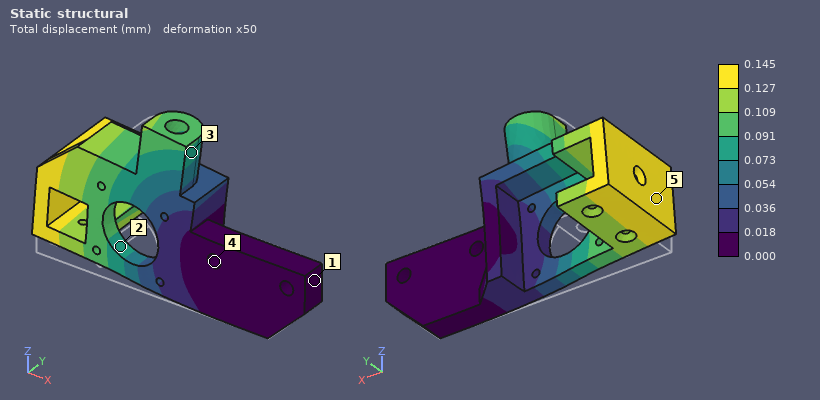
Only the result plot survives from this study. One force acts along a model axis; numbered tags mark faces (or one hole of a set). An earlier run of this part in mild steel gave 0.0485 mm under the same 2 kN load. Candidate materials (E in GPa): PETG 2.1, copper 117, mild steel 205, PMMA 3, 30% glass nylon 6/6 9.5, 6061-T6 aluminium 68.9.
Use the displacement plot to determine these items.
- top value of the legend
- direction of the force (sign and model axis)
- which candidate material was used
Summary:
0.145 mm
+Z
6061-T6 aluminium
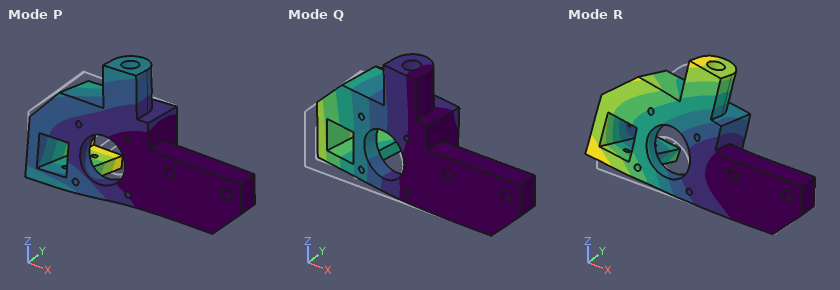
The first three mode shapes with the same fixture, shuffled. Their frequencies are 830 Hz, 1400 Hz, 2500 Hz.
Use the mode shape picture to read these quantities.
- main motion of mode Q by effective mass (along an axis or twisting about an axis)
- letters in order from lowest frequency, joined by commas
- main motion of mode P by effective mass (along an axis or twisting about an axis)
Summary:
along Y
Q, P, R
along Z
